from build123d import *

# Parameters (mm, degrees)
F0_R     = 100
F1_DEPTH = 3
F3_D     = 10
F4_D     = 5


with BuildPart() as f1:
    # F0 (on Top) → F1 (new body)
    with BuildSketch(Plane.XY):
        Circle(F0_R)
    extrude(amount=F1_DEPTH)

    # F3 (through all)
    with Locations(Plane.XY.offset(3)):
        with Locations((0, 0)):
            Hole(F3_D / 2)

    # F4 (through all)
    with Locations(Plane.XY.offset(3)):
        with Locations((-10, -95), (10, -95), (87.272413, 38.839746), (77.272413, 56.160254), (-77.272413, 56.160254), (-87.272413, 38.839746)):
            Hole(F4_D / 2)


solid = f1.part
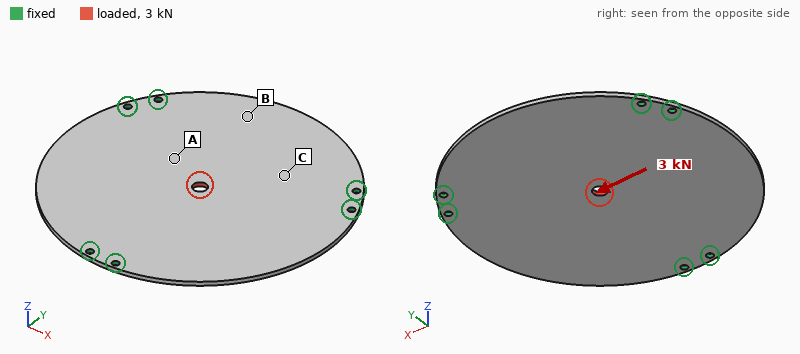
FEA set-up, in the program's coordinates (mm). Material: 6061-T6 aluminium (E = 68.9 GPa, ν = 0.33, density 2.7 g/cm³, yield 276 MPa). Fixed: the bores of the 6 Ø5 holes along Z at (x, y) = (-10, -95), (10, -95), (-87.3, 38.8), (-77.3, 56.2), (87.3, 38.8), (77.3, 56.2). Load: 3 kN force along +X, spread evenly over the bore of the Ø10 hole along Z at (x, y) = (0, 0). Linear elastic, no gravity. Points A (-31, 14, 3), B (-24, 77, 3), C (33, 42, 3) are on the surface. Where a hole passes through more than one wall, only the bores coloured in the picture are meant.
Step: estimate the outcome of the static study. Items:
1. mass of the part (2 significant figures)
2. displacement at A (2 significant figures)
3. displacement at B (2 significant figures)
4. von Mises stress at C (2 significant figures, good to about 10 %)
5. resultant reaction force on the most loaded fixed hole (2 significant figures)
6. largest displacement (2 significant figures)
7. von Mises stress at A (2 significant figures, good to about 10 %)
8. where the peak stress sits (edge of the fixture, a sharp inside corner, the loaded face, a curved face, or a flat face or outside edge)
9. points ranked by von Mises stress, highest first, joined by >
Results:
250 g
9.0 µm
3.5 µm
6.1 MPa
630 N
17 µm
10 MPa
the loaded face
A > C > B
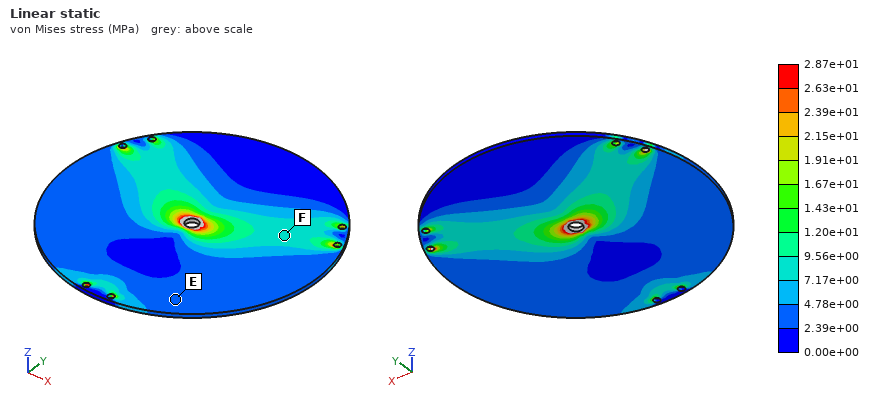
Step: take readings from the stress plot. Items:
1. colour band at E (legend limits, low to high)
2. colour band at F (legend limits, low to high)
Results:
2.39e+00 to 4.78e+00 MPa
7.17e+00 to 9.56e+00 MPa
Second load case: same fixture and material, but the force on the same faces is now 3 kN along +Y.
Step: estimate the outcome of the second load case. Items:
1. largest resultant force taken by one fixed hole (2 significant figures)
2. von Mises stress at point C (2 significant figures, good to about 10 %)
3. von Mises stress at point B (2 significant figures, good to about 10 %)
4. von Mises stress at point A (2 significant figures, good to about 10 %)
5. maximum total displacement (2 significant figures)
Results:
620 N
4.7 MPa
3.6 MPa
5.6 MPa
17 µm
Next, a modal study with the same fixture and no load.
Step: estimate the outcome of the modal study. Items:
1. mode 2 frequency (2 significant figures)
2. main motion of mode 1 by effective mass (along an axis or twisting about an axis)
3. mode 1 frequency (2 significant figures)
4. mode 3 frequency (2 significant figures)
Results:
530 Hz
along Z
500 Hz
530 Hz
